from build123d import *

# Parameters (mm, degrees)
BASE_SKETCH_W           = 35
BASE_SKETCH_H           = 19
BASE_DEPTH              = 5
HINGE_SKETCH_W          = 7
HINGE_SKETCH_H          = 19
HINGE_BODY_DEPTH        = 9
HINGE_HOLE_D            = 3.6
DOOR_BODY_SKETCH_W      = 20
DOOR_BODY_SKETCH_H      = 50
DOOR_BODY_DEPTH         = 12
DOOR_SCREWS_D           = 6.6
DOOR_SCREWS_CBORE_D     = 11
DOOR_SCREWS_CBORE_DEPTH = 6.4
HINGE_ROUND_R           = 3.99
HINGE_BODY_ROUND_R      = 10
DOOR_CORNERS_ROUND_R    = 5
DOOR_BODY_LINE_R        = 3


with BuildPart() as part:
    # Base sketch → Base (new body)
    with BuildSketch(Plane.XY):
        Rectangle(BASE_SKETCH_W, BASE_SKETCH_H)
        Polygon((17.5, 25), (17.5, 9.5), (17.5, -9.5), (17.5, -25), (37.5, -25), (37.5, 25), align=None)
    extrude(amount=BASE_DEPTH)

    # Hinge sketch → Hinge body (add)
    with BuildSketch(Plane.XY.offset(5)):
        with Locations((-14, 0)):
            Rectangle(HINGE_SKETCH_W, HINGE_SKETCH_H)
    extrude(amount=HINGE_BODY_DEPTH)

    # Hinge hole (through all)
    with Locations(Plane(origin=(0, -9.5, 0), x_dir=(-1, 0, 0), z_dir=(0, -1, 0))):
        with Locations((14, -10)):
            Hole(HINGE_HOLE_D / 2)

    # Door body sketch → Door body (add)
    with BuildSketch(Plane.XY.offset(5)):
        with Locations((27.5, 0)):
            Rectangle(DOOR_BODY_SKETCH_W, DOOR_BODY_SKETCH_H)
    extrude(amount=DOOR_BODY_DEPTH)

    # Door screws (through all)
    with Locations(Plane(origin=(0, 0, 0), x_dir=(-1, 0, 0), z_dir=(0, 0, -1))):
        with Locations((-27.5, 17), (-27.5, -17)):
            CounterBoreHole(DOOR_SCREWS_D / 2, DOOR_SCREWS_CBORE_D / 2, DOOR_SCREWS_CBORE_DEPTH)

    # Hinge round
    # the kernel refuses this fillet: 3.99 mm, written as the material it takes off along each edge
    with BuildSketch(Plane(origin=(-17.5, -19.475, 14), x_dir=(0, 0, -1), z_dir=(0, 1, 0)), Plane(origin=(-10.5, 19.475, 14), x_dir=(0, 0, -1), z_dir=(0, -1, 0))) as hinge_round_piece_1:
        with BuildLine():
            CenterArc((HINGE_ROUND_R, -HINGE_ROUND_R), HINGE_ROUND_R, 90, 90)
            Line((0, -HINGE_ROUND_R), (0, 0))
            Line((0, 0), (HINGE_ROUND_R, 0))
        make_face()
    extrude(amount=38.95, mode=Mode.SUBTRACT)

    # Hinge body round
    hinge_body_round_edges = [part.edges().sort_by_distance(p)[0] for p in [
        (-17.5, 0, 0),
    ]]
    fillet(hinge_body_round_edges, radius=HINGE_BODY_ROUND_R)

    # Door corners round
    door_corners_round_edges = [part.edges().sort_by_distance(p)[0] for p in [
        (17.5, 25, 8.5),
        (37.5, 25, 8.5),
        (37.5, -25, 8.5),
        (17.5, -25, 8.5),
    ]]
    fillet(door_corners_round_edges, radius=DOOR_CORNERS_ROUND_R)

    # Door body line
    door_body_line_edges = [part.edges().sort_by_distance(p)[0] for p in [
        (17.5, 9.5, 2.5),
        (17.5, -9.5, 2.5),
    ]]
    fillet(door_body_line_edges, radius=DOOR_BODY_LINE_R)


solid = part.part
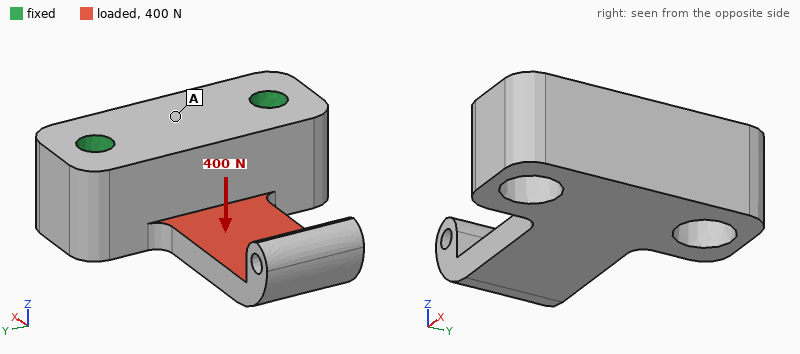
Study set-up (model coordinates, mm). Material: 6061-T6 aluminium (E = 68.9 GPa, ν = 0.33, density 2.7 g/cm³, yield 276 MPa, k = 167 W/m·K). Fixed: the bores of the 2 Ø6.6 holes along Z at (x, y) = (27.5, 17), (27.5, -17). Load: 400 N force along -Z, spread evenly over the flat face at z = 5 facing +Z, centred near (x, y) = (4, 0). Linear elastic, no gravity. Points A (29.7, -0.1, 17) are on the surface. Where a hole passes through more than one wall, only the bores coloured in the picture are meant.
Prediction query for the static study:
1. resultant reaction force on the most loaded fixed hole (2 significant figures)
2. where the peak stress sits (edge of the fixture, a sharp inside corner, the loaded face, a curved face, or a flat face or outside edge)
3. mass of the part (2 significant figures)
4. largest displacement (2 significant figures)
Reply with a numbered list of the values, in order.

1. 240 N
2. a curved face
3. 50 g
4. 0.15 mm
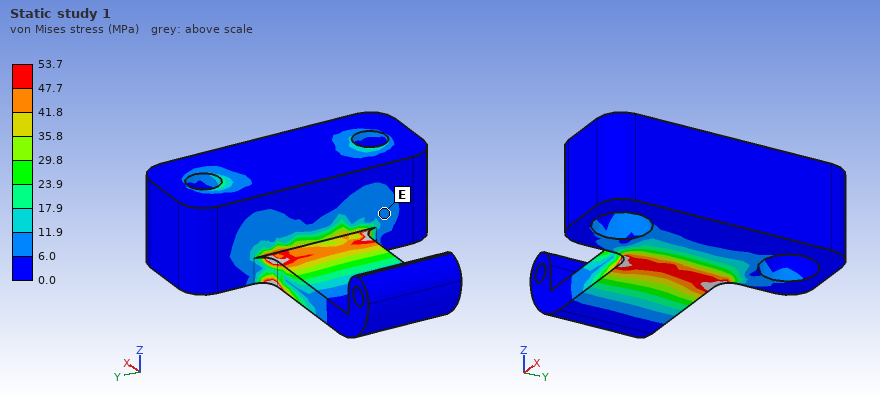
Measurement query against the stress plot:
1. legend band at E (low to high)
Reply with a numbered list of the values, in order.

1. 6.0 to 11.9 MPa
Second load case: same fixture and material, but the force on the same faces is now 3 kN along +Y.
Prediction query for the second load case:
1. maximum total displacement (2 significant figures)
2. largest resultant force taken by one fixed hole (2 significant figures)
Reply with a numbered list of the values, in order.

1. 0.20 mm
2. 2.6 kN
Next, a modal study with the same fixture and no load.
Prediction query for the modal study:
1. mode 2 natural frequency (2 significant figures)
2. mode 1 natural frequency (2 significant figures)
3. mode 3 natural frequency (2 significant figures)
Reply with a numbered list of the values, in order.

1. 6200 Hz
2. 2400 Hz
3. 10 kHz
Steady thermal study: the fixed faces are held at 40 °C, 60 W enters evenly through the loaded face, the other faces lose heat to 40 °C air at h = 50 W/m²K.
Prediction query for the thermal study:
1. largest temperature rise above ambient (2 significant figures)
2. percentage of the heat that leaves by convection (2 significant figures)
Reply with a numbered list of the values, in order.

1. 65 K
2. 9.3 %
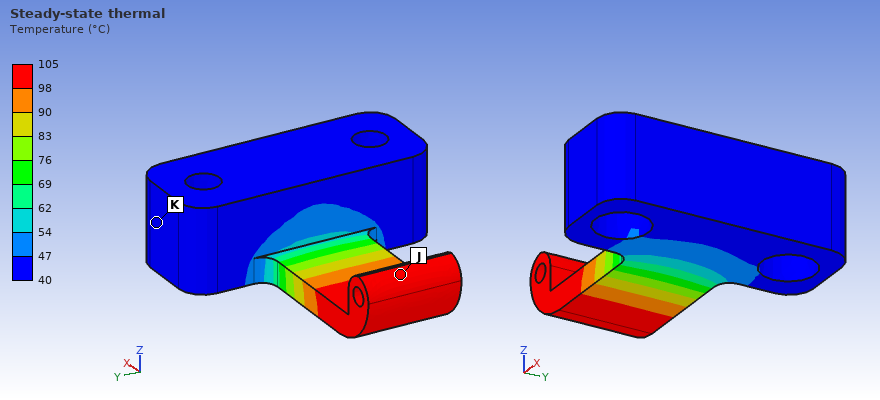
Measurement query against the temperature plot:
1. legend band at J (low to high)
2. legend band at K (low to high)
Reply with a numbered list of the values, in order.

1. 98 to 105 °C
2. 40 to 47 °C
